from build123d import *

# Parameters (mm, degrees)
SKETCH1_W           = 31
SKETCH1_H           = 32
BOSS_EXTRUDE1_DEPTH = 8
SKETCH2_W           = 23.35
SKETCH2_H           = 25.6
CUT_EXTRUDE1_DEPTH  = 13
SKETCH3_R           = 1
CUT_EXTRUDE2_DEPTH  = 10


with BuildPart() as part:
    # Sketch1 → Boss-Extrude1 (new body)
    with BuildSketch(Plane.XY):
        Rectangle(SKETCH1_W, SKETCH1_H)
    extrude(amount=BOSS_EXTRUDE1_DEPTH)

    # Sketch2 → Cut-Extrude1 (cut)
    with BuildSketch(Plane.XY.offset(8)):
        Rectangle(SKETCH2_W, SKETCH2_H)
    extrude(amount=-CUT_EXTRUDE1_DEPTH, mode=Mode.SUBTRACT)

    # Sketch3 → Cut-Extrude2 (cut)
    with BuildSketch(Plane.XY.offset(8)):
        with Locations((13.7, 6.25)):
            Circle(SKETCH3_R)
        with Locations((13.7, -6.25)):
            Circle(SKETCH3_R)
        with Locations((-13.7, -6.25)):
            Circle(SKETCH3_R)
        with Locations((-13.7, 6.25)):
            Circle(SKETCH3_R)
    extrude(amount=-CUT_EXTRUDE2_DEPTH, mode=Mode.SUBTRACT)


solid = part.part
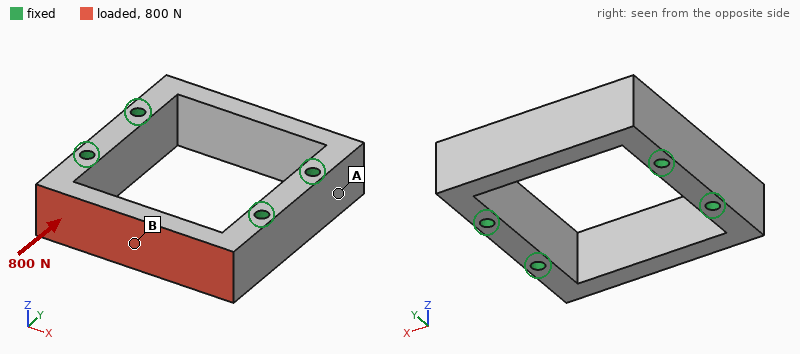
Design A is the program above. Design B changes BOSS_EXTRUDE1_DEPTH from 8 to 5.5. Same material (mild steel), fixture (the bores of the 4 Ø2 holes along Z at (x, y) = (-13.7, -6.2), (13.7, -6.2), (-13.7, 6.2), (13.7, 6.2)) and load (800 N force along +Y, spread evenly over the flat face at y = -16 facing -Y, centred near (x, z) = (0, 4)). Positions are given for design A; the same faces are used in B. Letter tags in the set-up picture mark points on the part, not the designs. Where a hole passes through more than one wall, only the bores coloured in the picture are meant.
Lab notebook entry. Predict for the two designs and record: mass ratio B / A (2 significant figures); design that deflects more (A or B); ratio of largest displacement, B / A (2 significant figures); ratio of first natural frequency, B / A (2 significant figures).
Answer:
0.69
B
1.5
0.85
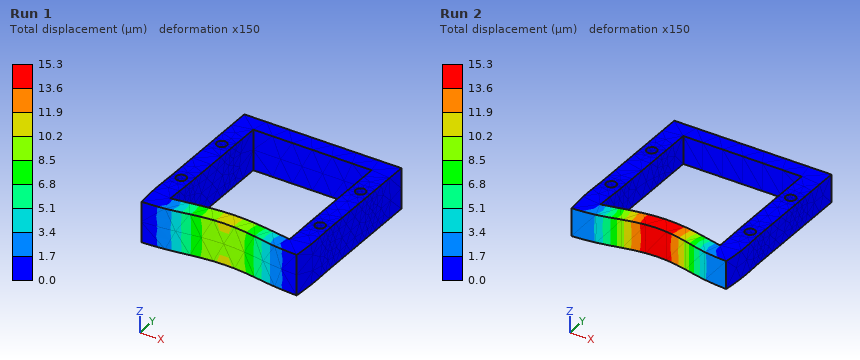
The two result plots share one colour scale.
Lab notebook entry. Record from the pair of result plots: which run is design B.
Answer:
Run 2
